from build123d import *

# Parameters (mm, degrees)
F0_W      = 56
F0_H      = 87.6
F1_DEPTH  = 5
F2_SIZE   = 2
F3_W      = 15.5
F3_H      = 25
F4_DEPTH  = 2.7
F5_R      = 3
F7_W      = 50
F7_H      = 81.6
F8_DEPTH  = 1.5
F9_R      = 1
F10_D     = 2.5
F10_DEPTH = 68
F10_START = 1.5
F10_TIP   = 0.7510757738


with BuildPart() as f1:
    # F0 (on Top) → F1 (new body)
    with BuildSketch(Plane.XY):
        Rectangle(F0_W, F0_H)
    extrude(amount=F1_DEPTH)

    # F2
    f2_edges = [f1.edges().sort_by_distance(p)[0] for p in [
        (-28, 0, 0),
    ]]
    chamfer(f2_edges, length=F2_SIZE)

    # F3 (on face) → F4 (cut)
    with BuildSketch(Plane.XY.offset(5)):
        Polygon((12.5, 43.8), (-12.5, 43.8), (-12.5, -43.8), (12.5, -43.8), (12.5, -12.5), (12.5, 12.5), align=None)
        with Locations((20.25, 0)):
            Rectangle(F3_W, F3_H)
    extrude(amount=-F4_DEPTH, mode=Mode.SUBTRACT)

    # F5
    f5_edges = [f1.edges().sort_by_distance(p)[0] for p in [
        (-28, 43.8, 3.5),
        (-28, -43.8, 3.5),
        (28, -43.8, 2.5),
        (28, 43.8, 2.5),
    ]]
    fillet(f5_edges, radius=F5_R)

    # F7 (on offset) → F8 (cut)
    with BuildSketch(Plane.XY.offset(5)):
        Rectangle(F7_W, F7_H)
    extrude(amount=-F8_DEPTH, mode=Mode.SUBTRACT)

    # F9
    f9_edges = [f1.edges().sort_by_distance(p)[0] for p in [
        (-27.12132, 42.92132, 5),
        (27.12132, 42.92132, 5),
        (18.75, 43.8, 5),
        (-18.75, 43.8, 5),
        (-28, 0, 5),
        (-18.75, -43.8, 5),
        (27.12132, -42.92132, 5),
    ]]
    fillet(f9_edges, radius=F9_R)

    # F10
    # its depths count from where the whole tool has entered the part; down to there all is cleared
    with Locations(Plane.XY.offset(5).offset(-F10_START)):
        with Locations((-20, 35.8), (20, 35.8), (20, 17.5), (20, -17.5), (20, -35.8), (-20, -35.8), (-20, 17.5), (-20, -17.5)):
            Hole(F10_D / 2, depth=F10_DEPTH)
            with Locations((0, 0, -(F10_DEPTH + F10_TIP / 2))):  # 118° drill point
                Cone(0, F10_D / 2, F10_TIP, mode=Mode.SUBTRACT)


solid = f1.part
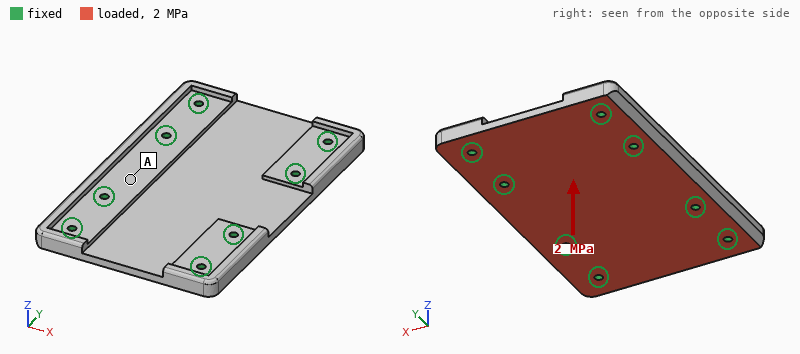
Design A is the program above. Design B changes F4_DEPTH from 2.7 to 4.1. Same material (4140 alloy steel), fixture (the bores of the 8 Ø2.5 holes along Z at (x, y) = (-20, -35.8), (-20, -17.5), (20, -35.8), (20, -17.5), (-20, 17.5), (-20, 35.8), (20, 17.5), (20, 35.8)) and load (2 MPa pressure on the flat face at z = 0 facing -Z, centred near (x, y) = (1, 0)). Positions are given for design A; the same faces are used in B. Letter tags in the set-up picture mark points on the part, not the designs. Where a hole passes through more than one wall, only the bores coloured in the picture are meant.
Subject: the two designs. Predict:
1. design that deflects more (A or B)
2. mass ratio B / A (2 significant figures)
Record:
B
0.75
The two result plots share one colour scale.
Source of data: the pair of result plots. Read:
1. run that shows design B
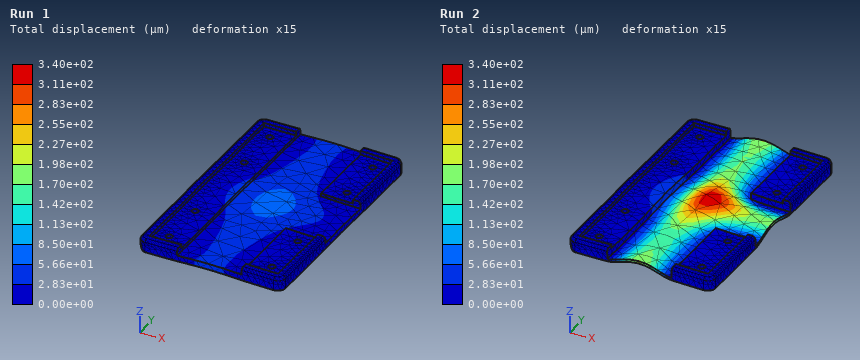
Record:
Run 2
